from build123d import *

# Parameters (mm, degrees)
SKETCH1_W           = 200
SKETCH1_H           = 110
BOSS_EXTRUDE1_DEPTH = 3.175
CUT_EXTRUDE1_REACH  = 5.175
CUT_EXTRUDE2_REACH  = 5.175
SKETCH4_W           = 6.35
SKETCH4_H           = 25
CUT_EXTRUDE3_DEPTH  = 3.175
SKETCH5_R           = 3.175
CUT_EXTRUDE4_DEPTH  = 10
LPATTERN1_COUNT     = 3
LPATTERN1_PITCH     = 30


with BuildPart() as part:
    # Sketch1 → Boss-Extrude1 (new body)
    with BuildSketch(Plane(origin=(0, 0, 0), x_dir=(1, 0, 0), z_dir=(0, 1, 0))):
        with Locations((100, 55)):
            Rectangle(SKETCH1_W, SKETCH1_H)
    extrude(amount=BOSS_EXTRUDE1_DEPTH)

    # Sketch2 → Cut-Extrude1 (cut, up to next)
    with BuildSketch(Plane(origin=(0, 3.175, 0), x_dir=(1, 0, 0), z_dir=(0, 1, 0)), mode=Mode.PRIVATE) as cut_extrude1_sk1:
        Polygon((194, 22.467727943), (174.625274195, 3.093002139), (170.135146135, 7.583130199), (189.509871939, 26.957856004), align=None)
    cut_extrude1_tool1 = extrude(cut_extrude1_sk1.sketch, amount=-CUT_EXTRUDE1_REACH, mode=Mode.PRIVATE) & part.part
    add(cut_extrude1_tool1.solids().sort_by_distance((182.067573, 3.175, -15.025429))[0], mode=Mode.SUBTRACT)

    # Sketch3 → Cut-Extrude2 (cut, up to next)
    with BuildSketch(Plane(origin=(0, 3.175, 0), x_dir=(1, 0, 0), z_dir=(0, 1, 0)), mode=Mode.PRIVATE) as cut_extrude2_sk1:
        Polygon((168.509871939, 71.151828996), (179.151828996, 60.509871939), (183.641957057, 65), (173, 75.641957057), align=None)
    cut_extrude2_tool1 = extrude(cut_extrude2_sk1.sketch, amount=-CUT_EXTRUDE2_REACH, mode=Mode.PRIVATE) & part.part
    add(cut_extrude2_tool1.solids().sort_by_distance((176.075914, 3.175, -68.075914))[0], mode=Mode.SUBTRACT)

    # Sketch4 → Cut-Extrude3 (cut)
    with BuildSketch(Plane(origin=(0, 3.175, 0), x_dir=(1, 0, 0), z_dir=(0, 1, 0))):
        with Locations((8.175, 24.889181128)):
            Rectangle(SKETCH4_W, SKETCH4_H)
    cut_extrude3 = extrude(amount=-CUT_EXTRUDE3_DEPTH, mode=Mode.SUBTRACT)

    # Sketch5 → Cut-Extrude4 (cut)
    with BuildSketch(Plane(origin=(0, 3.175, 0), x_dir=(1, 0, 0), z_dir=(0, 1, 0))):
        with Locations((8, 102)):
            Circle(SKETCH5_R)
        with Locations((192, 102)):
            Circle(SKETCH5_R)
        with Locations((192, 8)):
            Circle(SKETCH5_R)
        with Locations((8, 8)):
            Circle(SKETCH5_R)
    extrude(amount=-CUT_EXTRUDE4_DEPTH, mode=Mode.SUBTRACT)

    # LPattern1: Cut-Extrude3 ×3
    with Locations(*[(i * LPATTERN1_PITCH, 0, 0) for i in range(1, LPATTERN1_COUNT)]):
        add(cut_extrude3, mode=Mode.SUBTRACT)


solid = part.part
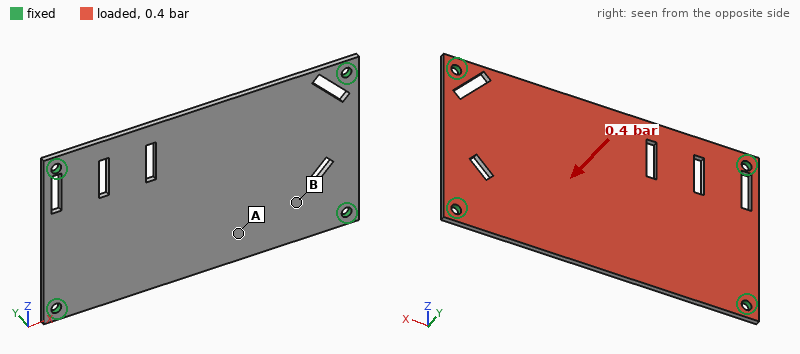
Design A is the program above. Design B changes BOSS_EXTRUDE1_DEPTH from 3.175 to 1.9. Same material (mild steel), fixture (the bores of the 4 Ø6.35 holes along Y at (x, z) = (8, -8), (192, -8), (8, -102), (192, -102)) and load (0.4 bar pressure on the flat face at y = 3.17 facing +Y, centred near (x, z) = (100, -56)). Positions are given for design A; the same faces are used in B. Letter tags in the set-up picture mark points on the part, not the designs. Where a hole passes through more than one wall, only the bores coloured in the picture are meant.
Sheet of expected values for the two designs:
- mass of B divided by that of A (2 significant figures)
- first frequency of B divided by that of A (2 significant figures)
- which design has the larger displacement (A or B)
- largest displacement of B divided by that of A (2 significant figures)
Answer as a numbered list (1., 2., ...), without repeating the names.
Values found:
1. 0.60
2. 0.61
3. B
4. 4.5
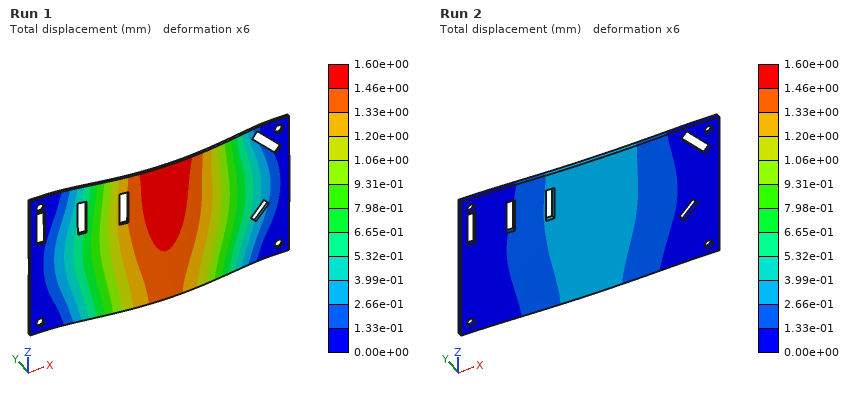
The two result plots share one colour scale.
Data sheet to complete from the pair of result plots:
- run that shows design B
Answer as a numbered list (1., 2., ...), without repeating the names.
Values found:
1. Run 1
